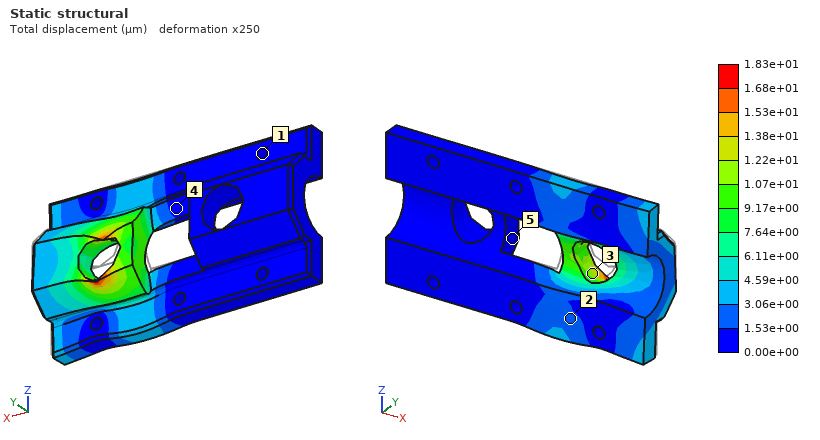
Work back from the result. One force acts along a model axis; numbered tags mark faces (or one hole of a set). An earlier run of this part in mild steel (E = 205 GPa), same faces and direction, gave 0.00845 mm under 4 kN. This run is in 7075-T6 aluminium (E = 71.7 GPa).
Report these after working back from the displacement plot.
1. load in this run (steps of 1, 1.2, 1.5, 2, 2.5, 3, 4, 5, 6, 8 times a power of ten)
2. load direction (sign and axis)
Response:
3 kN
-Z
